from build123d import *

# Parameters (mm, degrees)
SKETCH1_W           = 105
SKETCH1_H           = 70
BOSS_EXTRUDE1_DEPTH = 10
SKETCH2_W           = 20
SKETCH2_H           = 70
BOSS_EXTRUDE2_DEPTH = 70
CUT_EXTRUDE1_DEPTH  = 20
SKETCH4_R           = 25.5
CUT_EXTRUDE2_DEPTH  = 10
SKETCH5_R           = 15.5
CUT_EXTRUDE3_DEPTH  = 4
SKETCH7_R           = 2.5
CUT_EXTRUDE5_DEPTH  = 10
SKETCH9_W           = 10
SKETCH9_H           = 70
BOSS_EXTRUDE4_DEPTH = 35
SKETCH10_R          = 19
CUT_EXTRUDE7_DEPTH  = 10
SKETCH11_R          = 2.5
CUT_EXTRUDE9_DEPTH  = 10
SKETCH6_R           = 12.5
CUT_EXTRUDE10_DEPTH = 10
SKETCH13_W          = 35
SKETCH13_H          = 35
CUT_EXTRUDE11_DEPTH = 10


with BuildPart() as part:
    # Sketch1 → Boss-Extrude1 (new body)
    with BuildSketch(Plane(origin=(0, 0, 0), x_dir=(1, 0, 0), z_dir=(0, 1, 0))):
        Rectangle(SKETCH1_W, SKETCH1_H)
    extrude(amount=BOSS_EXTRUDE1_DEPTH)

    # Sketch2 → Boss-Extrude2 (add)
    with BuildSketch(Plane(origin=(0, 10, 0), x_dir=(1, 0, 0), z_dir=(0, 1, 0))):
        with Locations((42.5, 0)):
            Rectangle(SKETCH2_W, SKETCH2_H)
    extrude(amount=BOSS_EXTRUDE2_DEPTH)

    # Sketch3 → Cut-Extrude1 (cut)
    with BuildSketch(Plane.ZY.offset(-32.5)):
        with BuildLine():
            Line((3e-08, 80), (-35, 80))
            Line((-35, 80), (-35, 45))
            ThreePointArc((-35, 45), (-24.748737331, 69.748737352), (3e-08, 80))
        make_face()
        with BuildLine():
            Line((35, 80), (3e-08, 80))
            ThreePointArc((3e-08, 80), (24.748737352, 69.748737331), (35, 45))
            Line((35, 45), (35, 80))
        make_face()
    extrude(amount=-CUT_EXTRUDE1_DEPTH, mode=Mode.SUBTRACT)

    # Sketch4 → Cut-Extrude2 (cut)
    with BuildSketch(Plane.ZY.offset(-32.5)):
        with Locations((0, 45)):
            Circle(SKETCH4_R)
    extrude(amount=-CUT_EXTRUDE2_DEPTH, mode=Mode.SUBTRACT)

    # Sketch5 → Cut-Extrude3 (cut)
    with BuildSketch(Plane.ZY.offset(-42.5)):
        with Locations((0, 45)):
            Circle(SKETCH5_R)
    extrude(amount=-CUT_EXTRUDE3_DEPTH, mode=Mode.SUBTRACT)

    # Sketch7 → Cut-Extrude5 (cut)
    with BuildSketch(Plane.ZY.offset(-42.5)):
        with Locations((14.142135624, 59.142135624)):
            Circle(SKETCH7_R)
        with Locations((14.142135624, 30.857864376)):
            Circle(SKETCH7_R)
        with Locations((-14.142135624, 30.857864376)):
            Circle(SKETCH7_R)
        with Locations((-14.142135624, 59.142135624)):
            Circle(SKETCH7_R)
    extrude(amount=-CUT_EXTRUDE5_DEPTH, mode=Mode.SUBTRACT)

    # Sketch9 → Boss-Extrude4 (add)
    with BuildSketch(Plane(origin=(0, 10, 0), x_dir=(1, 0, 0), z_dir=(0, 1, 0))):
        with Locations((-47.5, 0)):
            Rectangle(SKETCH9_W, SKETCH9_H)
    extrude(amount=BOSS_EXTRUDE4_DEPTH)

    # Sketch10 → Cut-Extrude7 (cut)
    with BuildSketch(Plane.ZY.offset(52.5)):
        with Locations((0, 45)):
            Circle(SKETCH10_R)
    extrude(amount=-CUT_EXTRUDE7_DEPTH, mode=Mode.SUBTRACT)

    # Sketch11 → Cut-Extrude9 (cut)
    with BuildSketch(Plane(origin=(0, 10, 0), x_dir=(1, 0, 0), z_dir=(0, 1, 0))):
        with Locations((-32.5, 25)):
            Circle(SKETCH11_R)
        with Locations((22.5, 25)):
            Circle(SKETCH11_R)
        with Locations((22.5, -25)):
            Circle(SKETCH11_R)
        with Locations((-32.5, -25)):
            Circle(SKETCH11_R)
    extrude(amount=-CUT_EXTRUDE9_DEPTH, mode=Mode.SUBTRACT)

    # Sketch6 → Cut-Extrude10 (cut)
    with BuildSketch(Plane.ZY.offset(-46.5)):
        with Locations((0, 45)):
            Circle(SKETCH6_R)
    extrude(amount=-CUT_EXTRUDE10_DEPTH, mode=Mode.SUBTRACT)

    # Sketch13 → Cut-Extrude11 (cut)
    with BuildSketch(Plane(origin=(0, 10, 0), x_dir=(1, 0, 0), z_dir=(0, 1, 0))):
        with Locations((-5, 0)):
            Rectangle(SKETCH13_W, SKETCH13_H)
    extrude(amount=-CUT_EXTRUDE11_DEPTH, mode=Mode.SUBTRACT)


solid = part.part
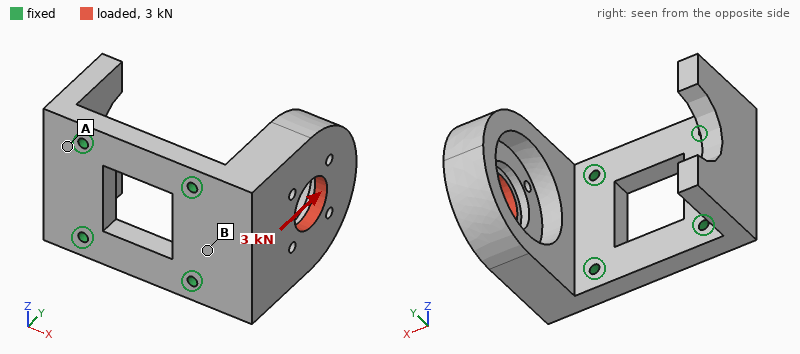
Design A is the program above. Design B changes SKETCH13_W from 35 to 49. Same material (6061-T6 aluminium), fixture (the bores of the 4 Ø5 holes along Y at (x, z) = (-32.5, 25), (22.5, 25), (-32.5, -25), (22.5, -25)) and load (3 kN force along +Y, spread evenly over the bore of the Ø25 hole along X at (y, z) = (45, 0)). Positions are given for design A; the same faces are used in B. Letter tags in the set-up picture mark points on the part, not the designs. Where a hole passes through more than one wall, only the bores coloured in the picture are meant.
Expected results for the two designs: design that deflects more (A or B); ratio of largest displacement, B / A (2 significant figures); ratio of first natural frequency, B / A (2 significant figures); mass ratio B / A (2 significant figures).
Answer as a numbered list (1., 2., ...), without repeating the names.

1. B
2. 1.1
3. 0.94
4. 0.96
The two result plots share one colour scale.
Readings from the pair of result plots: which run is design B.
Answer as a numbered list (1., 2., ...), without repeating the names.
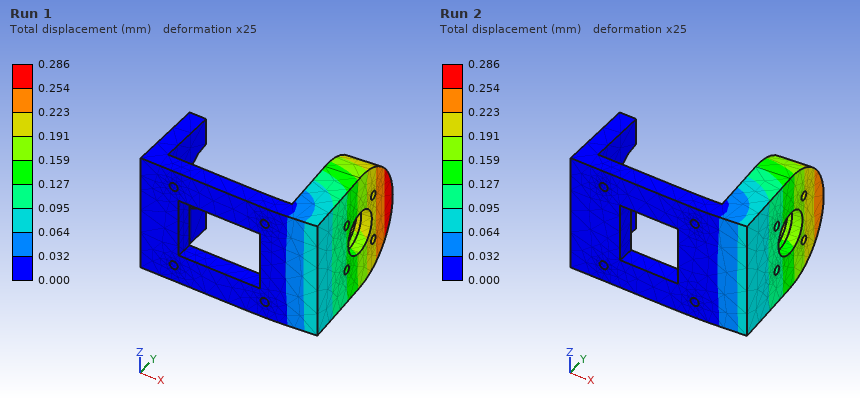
1. Run 1
